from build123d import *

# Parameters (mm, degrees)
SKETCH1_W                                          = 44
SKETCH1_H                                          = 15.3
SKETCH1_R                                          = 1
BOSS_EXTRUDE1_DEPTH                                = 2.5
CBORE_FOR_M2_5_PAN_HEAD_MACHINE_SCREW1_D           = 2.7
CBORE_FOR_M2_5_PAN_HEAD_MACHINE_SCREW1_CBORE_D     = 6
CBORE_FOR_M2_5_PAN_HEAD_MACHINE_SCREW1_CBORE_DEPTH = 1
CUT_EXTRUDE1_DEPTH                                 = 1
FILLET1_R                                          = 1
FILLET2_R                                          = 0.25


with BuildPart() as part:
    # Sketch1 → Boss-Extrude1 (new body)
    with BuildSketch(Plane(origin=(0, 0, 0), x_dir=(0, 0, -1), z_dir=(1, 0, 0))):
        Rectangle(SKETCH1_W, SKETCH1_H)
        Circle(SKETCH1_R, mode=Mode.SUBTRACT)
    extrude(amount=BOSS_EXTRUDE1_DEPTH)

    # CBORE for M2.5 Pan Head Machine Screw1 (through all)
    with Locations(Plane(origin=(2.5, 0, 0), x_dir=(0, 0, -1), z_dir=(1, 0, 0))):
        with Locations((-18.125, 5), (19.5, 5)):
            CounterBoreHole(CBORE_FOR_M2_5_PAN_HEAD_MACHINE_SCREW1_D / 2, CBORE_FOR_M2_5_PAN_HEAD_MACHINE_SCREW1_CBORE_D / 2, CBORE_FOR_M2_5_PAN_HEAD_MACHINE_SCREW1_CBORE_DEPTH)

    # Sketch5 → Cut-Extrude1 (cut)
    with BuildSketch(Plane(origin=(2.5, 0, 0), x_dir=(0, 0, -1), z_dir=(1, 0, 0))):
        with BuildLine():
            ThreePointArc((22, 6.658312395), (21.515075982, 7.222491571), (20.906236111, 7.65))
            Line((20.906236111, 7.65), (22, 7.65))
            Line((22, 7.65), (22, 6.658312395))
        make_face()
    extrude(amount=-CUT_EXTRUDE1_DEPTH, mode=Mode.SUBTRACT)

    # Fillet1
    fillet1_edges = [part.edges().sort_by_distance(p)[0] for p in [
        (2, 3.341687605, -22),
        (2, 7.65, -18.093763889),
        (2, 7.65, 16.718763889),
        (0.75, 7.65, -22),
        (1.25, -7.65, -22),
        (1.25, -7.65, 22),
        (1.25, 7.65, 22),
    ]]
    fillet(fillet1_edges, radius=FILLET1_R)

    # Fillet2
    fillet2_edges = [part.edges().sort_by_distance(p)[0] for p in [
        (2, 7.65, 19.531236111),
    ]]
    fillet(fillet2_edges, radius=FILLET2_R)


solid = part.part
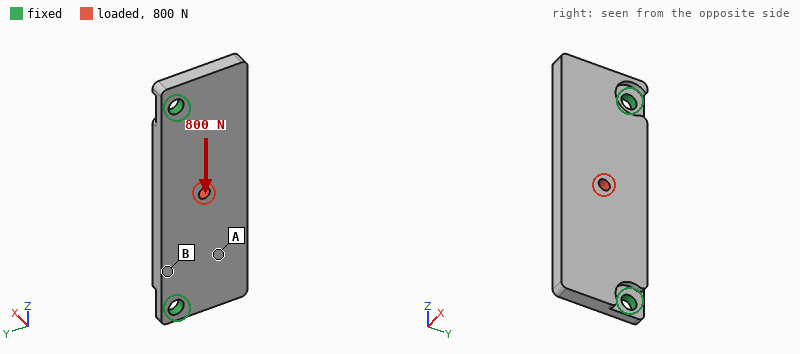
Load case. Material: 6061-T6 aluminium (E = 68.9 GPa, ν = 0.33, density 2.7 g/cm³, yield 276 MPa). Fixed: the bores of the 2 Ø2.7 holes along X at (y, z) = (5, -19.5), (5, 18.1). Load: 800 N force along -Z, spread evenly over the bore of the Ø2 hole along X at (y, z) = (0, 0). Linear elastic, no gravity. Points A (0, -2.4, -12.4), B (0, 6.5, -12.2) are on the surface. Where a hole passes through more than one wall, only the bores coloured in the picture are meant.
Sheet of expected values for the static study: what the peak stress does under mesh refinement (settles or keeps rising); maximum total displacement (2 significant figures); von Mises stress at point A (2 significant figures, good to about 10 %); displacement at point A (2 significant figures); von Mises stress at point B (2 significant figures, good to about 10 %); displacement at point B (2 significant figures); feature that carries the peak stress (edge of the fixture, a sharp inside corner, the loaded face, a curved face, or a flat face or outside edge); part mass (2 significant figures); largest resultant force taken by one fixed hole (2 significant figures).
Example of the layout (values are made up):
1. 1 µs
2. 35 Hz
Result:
1. keeps rising
2. 7.8 µm
3. 12 MPa
4. 5.1 µm
5. 28 MPa
6. 3.5 µm
7. edge of the fixture
8. 4.3 g
9. 420 N
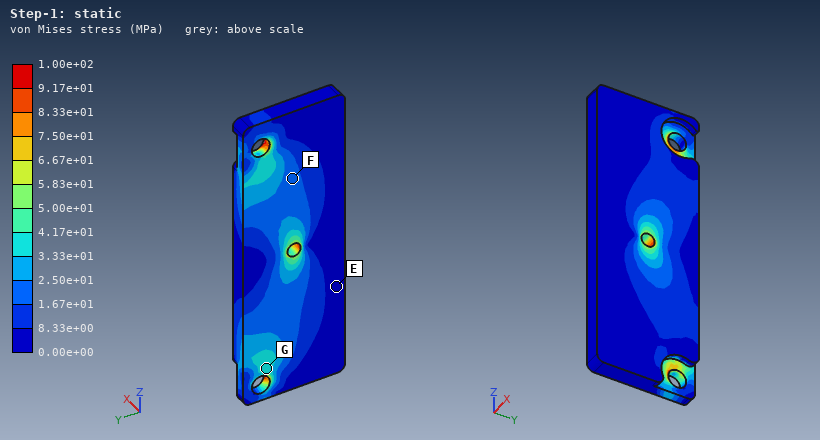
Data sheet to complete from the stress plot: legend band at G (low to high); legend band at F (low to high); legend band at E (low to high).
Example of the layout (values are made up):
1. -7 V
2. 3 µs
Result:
1. 3.33e+01 to 4.17e+01 MPa
2. 1.67e+01 to 2.50e+01 MPa
3. 0.00e+00 to 8.33e+00 MPa
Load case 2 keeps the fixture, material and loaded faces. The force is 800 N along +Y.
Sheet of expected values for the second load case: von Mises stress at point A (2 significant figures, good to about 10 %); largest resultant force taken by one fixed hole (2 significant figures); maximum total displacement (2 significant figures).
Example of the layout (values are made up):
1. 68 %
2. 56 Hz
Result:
1. 27 MPa
2. 520 N
3. 34 µm
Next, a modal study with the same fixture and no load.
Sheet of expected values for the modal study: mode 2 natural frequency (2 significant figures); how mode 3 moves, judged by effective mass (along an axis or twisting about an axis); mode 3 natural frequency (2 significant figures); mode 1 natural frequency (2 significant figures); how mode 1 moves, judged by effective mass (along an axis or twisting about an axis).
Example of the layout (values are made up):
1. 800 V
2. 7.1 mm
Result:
1. 9200 Hz
2. twisting about Y
3. 11 kHz
4. 4700 Hz
5. along X
